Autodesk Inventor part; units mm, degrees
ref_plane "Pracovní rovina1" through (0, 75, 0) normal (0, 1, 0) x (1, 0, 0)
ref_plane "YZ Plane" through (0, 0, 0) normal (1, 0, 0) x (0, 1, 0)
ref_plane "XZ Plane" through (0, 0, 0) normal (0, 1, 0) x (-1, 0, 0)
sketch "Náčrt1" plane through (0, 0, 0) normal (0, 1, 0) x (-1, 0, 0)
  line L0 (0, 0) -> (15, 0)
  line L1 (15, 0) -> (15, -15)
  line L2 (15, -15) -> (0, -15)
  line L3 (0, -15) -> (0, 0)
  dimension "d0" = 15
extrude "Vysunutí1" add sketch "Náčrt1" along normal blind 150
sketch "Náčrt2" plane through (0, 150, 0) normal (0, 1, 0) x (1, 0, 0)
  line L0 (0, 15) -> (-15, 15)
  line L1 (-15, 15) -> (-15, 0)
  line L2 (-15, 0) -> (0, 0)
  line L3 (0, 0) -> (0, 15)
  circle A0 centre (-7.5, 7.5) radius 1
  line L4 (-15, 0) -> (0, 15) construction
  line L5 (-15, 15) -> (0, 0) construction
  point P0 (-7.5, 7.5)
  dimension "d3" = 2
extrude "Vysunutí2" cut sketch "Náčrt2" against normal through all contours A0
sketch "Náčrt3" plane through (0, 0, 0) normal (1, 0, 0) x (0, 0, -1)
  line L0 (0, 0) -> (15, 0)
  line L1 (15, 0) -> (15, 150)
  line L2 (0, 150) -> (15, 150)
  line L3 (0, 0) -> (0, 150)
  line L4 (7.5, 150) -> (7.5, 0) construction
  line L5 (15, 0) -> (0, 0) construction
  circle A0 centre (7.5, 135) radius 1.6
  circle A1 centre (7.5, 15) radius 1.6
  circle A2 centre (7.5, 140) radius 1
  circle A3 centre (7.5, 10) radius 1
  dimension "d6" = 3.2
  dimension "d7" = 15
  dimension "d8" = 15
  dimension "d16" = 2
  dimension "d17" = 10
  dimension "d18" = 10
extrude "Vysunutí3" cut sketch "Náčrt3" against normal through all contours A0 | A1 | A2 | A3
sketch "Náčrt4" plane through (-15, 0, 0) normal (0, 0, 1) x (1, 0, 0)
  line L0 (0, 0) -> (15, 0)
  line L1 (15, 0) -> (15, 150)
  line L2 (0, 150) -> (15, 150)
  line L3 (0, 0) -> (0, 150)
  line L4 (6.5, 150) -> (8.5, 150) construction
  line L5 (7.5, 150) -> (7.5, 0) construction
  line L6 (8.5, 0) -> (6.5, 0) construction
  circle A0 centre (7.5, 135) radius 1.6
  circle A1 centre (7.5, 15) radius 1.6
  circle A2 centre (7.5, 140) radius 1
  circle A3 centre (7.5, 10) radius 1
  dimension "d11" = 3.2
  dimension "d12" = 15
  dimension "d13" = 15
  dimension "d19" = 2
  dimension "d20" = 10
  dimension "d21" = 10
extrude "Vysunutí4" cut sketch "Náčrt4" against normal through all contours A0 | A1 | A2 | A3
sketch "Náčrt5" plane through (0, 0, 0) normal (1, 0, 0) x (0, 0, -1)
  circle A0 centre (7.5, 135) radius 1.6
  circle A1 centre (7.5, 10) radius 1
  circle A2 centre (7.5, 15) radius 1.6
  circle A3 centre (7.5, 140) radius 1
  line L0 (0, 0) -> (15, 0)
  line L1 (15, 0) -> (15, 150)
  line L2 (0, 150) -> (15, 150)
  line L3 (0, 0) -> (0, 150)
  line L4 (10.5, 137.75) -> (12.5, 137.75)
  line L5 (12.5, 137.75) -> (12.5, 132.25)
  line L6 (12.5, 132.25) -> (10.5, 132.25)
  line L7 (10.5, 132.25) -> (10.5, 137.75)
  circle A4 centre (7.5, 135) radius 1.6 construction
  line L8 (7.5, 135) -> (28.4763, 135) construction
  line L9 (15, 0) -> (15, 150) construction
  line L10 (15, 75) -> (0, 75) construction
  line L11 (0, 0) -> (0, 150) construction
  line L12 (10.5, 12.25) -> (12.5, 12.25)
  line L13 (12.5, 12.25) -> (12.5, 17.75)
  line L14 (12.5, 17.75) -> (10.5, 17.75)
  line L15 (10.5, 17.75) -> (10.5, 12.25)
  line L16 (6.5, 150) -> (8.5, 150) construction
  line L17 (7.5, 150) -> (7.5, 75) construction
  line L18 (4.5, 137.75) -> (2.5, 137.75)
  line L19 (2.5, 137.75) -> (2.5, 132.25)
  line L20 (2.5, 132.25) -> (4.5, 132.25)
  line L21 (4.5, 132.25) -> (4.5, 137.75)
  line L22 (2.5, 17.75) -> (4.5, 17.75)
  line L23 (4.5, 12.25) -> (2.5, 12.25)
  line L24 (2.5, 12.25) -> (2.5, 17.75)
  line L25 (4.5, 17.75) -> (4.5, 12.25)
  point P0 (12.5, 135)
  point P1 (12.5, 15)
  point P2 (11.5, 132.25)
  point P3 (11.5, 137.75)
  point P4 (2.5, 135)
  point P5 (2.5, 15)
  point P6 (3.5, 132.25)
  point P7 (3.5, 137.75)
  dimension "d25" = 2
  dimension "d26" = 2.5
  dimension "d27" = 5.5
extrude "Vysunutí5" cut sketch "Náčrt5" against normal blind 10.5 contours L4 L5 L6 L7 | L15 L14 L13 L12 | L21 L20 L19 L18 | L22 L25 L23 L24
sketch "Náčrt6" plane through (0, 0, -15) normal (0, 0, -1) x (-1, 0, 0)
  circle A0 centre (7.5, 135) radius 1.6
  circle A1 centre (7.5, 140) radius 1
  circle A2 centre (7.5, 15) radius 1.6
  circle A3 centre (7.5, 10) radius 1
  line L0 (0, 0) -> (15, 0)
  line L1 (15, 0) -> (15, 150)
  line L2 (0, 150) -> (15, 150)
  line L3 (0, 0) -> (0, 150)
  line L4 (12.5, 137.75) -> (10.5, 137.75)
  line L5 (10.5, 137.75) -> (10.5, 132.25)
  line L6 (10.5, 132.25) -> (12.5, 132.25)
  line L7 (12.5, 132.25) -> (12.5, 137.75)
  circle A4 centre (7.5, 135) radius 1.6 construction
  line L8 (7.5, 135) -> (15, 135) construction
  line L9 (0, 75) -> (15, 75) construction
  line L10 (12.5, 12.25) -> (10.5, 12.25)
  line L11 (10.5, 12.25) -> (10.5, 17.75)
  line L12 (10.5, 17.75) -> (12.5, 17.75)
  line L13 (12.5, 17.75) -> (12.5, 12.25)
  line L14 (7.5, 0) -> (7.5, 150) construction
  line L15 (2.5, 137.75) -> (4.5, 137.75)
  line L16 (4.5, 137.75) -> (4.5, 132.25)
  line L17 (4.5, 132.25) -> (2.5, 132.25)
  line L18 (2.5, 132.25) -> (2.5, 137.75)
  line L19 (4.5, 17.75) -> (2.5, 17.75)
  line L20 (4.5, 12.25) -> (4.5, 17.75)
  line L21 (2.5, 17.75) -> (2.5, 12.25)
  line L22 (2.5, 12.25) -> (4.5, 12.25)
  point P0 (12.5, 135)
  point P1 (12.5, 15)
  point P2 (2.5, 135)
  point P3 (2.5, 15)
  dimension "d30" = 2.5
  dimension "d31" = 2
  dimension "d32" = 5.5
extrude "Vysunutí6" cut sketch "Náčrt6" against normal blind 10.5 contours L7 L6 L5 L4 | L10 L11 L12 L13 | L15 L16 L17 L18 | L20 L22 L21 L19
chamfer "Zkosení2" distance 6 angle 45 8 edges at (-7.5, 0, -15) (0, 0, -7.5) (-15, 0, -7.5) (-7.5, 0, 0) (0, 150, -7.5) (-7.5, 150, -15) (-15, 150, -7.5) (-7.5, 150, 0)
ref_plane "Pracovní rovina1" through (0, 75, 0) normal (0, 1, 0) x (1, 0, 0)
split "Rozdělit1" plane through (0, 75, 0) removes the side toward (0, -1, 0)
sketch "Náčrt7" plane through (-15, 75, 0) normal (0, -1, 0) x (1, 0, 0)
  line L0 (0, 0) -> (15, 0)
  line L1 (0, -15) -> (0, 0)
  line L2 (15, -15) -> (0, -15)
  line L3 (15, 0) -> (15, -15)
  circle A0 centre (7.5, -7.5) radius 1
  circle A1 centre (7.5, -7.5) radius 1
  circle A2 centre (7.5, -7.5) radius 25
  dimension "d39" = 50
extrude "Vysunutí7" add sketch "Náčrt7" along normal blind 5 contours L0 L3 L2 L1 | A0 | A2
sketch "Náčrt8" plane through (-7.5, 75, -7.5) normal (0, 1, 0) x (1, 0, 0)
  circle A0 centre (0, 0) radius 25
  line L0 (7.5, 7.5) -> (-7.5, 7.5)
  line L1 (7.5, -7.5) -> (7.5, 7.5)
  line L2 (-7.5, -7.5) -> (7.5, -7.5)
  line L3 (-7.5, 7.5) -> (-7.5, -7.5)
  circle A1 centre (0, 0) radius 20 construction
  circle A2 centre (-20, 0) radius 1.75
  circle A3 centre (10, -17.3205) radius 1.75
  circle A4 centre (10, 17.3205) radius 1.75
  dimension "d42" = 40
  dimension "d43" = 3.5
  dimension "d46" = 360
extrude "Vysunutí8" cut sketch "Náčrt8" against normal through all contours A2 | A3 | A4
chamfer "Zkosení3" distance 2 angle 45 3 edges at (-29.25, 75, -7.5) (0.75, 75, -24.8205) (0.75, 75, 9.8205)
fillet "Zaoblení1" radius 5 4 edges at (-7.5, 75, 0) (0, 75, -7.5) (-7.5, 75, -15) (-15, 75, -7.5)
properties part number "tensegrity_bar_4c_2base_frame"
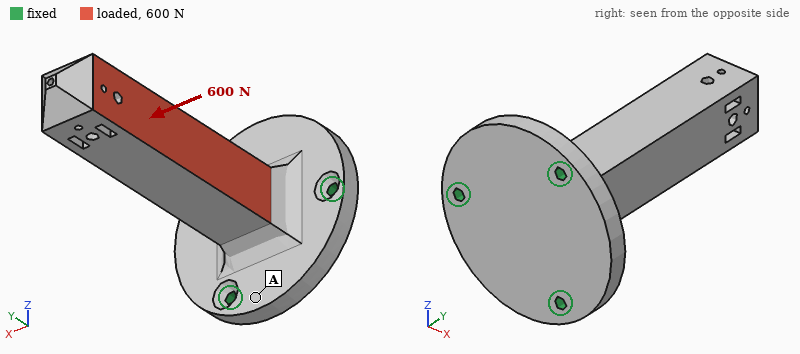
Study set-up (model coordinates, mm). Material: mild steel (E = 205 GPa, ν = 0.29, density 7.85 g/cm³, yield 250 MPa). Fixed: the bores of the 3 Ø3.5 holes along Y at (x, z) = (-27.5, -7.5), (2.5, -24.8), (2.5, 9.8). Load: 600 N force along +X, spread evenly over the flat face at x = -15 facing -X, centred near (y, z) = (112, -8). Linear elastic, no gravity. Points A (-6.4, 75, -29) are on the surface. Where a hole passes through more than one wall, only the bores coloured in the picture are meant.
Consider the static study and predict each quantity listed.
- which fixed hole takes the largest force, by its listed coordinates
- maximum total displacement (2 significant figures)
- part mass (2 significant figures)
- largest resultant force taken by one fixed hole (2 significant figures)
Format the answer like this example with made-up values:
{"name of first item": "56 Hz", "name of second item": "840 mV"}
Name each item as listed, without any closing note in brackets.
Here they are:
{"which fixed hole takes the largest force, by its listed coordinates": "(-27.5, -7.5)", "maximum total displacement": "61 µm", "part mass": "200 g", "largest resultant force taken by one fixed hole": "950 N"}
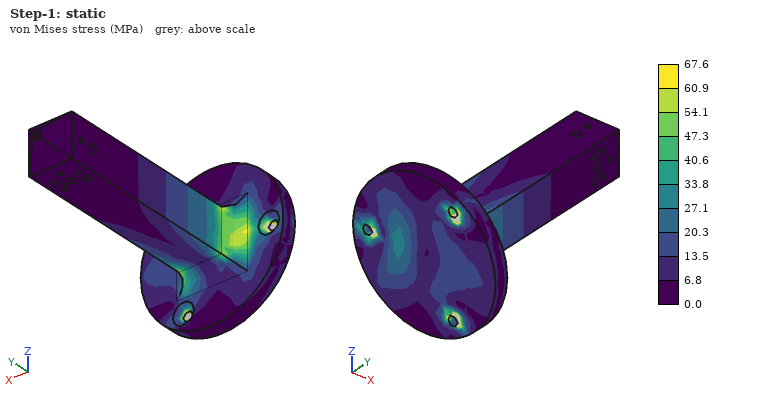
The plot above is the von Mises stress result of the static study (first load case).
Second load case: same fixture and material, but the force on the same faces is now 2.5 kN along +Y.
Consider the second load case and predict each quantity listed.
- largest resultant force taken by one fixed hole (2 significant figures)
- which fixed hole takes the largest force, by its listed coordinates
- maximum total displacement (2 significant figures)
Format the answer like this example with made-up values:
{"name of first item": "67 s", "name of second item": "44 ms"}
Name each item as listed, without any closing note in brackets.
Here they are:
{"largest resultant force taken by one fixed hole": "1.7 kN", "which fixed hole takes the largest force, by its listed coordinates": "(-27.5, -7.5)", "maximum total displacement": "65 µm"}
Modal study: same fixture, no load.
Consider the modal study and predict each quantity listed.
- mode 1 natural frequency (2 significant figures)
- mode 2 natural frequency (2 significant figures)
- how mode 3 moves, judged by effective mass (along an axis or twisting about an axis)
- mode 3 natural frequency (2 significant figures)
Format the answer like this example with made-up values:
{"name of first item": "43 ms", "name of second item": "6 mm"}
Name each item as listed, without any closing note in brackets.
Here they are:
{"mode 1 natural frequency": "1900 Hz", "mode 2 natural frequency": "1900 Hz", "how mode 3 moves, judged by effective mass": "along Y", "mode 3 natural frequency": "8000 Hz"}
